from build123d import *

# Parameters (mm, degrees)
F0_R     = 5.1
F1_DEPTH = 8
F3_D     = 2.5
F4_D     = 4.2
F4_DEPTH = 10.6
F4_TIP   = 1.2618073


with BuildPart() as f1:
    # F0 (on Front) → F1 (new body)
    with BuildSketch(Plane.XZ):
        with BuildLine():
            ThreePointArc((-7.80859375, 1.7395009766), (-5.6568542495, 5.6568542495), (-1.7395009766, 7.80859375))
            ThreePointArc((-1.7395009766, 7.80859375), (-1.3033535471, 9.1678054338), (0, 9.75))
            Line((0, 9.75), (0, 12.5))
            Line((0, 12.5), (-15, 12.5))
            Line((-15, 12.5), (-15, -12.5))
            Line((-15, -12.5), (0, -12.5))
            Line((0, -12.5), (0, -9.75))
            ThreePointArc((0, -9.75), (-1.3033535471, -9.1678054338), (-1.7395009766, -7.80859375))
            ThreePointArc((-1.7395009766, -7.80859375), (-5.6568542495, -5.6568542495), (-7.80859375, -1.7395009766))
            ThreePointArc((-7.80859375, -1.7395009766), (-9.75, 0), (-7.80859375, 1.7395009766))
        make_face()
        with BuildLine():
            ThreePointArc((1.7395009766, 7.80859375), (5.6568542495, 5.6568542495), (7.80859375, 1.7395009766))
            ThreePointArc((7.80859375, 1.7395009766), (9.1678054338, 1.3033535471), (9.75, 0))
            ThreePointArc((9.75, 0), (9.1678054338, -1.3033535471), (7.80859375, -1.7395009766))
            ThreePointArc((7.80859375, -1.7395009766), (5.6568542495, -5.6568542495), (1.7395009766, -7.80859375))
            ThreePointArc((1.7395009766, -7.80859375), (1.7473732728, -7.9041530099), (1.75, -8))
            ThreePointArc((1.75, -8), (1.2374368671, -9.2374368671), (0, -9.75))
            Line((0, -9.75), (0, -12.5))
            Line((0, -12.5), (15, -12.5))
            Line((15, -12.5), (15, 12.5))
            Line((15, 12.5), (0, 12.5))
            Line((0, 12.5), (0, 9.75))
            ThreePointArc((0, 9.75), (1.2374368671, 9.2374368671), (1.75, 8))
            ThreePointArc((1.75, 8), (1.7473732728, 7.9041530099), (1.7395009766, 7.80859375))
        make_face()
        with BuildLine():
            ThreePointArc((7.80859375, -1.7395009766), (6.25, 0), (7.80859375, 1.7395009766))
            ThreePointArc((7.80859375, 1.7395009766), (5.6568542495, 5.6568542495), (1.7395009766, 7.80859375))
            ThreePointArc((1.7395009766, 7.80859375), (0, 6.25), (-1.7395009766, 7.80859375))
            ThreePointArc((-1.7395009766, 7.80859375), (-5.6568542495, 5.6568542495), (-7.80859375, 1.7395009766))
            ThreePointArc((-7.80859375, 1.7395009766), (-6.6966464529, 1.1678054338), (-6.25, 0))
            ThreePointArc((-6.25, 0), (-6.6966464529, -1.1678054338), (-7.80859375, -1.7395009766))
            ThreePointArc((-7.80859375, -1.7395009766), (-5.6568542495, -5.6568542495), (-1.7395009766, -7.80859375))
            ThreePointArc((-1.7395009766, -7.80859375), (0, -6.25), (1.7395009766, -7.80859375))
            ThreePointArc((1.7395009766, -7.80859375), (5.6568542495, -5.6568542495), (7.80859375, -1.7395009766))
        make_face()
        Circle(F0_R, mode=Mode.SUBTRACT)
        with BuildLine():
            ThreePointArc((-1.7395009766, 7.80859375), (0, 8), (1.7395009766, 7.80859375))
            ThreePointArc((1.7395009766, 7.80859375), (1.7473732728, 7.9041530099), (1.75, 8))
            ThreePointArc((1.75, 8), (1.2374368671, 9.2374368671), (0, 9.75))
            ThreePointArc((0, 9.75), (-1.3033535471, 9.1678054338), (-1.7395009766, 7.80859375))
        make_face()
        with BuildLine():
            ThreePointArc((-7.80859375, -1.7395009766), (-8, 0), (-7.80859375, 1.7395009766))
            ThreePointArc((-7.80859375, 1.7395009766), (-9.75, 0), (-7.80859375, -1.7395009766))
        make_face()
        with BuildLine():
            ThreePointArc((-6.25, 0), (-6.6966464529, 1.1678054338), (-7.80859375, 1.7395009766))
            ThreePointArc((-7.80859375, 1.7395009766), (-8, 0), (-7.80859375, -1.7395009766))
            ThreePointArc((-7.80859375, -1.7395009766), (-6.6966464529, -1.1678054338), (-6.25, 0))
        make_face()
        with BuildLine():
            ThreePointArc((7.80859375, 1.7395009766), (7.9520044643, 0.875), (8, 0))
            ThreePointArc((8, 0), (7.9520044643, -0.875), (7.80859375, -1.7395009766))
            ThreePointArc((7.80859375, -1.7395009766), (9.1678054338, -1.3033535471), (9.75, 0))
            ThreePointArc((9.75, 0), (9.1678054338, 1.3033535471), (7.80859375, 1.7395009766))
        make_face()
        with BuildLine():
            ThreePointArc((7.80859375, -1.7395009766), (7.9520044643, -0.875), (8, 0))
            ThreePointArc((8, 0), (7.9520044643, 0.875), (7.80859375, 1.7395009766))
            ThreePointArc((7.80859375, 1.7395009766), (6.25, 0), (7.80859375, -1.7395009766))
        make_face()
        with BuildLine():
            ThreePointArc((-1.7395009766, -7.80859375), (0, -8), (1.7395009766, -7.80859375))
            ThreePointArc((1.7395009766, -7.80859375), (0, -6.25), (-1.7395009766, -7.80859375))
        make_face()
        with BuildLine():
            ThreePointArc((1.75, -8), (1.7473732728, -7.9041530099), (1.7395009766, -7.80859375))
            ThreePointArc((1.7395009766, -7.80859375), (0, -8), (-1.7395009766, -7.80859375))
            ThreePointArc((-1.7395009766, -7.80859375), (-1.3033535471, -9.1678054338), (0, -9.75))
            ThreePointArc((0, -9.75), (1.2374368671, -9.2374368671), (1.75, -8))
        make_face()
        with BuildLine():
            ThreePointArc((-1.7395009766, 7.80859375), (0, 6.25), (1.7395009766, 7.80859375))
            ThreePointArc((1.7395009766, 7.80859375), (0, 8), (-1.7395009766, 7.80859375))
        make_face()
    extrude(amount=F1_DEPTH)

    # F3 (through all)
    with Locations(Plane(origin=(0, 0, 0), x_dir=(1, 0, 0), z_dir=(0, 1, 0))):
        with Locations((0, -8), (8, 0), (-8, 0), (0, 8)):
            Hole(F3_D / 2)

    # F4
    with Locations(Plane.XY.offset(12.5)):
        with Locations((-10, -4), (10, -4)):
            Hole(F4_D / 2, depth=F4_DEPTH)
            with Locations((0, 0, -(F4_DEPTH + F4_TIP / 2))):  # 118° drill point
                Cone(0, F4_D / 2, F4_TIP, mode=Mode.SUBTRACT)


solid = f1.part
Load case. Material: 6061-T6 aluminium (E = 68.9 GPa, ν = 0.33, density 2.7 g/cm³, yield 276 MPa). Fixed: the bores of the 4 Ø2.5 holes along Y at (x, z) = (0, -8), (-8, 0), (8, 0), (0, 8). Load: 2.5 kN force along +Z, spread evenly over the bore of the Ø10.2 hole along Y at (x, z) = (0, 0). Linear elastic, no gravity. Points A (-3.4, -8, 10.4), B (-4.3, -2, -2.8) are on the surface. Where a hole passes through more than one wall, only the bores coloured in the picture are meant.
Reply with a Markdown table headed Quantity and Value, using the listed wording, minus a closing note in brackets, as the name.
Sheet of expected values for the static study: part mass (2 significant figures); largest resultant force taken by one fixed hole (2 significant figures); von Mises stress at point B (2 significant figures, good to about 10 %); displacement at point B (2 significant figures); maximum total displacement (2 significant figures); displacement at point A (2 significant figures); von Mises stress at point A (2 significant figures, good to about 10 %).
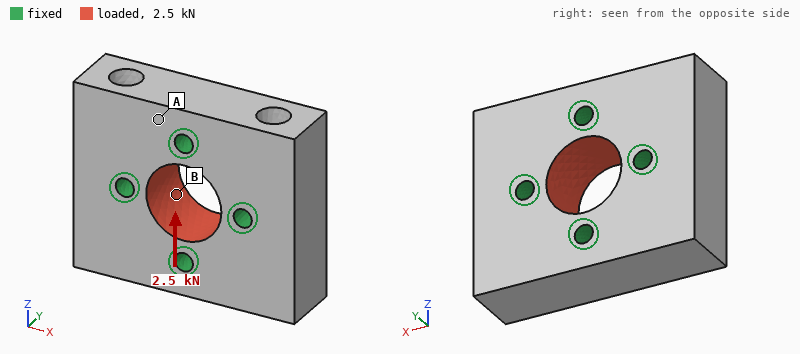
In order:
| Quantity | Value |
|---|---|
| part mass | 13 g |
| largest resultant force taken by one fixed hole | 640 N |
| von Mises stress at point B | 13 MPa |
| displacement at point B | 0.93 µm |
| maximum total displacement | 1.0 µm |
| displacement at point A | 0.30 µm |
| von Mises stress at point A | 4.0 MPa |
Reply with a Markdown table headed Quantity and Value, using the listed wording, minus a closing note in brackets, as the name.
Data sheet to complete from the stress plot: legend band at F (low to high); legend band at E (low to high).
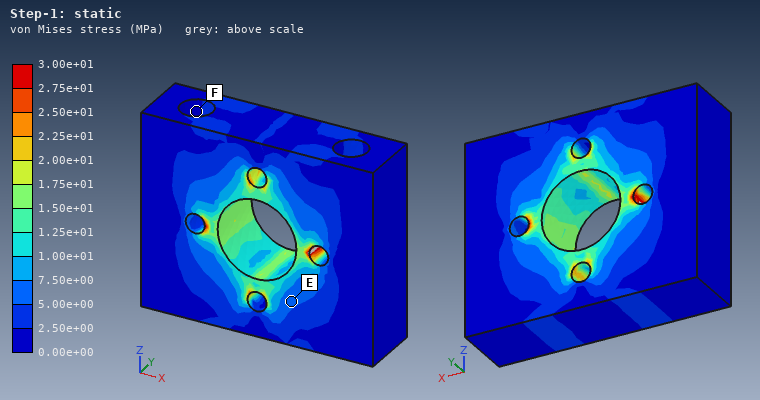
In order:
| Quantity | Value |
|---|---|
| legend band at F | 0.00e+00 to 2.50e+00 MPa |
| legend band at E | 5.00e+00 to 7.50e+00 MPa |
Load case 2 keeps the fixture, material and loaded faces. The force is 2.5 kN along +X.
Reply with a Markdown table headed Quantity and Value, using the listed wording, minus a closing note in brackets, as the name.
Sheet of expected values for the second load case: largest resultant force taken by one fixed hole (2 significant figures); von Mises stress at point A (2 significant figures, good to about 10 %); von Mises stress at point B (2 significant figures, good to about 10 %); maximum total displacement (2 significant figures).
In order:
| Quantity | Value |
|---|---|
| largest resultant force taken by one fixed hole | 630 N |
| von Mises stress at point A | 2.8 MPa |
| von Mises stress at point B | 11 MPa |
| maximum total displacement | 1.0 µm |
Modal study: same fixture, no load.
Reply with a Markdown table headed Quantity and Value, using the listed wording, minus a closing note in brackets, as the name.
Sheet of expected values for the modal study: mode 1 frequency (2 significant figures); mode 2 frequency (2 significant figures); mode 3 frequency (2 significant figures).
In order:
| Quantity | Value |
|---|---|
| mode 1 frequency | 39 kHz |
| mode 2 frequency | 40 kHz |
| mode 3 frequency | 41 kHz |
